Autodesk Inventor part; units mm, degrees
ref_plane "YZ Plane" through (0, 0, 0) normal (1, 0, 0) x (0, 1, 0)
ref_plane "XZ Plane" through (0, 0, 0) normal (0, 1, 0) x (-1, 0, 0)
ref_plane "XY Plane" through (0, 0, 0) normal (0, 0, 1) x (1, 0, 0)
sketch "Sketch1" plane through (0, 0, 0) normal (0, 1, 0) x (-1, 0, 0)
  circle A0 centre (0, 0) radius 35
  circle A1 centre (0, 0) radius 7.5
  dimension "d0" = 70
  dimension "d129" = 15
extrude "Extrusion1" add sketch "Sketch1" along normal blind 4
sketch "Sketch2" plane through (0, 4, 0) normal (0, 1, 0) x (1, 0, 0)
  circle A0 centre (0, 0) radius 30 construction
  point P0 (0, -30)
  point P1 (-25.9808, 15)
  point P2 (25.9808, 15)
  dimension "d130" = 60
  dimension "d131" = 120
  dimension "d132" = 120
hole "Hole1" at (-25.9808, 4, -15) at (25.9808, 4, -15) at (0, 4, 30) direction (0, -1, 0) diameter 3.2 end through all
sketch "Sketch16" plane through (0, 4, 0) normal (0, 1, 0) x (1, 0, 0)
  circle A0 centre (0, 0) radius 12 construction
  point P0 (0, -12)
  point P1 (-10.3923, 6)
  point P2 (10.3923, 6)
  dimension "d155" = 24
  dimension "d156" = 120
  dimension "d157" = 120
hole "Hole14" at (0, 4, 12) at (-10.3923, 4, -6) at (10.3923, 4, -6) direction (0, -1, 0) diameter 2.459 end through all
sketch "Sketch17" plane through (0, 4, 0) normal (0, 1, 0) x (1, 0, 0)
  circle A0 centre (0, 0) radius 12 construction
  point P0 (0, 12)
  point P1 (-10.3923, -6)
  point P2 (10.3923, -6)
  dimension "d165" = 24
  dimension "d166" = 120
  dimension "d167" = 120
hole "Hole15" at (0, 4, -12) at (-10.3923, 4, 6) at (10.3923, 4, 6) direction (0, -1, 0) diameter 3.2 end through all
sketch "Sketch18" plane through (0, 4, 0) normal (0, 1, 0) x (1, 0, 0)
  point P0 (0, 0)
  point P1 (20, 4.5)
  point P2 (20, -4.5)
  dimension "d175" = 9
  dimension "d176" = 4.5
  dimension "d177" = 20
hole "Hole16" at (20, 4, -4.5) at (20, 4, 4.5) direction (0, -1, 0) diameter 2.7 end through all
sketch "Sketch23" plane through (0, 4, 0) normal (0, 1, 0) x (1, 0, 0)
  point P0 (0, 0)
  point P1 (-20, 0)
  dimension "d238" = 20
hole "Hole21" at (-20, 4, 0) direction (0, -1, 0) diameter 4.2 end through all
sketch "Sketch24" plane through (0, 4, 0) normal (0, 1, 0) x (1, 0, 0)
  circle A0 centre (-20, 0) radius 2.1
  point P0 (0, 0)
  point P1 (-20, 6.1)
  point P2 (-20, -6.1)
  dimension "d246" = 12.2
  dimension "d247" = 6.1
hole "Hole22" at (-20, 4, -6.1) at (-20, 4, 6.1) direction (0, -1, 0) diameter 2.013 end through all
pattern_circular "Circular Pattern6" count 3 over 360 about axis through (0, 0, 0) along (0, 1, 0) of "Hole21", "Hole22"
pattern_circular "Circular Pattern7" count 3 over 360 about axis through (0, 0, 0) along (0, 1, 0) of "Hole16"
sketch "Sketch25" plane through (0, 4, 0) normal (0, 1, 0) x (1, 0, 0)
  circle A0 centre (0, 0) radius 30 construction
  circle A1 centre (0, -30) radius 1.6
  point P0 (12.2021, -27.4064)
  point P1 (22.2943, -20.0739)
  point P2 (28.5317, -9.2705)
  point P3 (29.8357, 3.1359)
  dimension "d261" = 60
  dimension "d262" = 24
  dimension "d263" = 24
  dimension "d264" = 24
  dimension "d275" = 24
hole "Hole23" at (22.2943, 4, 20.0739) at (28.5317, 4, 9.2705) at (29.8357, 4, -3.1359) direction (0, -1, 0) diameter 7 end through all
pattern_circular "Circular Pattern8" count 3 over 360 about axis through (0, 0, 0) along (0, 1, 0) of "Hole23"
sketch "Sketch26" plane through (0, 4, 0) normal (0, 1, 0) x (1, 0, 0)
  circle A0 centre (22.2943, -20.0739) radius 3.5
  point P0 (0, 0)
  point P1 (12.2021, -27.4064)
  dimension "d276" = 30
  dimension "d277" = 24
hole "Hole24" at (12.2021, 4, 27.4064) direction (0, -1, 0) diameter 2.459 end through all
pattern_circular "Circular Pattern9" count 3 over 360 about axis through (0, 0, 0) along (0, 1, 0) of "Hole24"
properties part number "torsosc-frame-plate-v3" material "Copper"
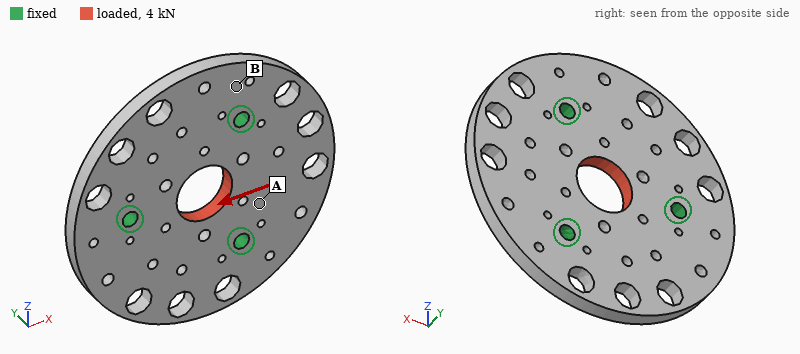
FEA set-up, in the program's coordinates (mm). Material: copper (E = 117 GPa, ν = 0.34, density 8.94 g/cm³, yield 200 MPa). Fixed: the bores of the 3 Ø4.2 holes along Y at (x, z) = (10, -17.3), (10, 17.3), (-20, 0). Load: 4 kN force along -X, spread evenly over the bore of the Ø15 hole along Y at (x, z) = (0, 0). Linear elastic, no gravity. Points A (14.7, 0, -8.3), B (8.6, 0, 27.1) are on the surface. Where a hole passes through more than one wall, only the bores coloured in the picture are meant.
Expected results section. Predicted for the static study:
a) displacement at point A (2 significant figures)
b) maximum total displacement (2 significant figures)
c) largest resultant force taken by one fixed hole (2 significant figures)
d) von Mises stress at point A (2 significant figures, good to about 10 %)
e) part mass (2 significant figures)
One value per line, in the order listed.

2.9 µm
5.5 µm
1.3 kN
16 MPa
110 g
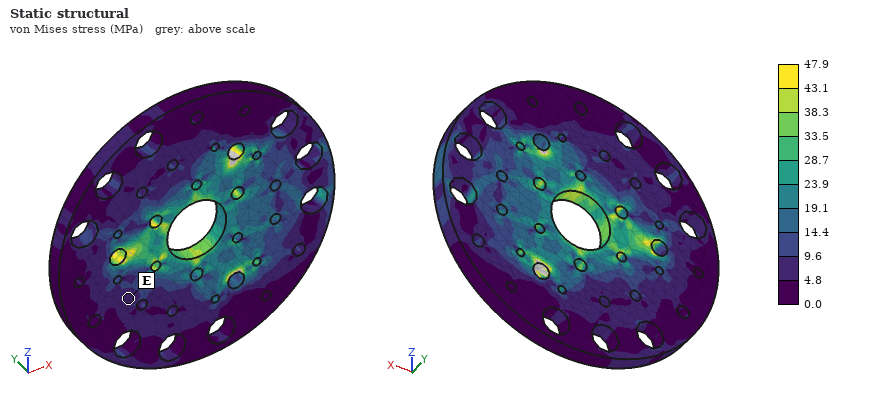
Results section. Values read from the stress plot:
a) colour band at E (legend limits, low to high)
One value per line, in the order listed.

4.8 to 9.6 MPa
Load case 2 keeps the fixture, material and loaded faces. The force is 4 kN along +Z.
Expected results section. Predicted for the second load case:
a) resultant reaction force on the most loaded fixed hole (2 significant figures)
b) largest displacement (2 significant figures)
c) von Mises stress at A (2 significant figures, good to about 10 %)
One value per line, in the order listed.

1.3 kN
5.3 µm
11 MPa
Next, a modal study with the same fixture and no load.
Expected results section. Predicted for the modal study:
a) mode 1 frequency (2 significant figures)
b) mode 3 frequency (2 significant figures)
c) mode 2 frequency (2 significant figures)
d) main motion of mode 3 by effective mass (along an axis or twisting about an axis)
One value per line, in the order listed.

4200 Hz
4700 Hz
4200 Hz
along Y
